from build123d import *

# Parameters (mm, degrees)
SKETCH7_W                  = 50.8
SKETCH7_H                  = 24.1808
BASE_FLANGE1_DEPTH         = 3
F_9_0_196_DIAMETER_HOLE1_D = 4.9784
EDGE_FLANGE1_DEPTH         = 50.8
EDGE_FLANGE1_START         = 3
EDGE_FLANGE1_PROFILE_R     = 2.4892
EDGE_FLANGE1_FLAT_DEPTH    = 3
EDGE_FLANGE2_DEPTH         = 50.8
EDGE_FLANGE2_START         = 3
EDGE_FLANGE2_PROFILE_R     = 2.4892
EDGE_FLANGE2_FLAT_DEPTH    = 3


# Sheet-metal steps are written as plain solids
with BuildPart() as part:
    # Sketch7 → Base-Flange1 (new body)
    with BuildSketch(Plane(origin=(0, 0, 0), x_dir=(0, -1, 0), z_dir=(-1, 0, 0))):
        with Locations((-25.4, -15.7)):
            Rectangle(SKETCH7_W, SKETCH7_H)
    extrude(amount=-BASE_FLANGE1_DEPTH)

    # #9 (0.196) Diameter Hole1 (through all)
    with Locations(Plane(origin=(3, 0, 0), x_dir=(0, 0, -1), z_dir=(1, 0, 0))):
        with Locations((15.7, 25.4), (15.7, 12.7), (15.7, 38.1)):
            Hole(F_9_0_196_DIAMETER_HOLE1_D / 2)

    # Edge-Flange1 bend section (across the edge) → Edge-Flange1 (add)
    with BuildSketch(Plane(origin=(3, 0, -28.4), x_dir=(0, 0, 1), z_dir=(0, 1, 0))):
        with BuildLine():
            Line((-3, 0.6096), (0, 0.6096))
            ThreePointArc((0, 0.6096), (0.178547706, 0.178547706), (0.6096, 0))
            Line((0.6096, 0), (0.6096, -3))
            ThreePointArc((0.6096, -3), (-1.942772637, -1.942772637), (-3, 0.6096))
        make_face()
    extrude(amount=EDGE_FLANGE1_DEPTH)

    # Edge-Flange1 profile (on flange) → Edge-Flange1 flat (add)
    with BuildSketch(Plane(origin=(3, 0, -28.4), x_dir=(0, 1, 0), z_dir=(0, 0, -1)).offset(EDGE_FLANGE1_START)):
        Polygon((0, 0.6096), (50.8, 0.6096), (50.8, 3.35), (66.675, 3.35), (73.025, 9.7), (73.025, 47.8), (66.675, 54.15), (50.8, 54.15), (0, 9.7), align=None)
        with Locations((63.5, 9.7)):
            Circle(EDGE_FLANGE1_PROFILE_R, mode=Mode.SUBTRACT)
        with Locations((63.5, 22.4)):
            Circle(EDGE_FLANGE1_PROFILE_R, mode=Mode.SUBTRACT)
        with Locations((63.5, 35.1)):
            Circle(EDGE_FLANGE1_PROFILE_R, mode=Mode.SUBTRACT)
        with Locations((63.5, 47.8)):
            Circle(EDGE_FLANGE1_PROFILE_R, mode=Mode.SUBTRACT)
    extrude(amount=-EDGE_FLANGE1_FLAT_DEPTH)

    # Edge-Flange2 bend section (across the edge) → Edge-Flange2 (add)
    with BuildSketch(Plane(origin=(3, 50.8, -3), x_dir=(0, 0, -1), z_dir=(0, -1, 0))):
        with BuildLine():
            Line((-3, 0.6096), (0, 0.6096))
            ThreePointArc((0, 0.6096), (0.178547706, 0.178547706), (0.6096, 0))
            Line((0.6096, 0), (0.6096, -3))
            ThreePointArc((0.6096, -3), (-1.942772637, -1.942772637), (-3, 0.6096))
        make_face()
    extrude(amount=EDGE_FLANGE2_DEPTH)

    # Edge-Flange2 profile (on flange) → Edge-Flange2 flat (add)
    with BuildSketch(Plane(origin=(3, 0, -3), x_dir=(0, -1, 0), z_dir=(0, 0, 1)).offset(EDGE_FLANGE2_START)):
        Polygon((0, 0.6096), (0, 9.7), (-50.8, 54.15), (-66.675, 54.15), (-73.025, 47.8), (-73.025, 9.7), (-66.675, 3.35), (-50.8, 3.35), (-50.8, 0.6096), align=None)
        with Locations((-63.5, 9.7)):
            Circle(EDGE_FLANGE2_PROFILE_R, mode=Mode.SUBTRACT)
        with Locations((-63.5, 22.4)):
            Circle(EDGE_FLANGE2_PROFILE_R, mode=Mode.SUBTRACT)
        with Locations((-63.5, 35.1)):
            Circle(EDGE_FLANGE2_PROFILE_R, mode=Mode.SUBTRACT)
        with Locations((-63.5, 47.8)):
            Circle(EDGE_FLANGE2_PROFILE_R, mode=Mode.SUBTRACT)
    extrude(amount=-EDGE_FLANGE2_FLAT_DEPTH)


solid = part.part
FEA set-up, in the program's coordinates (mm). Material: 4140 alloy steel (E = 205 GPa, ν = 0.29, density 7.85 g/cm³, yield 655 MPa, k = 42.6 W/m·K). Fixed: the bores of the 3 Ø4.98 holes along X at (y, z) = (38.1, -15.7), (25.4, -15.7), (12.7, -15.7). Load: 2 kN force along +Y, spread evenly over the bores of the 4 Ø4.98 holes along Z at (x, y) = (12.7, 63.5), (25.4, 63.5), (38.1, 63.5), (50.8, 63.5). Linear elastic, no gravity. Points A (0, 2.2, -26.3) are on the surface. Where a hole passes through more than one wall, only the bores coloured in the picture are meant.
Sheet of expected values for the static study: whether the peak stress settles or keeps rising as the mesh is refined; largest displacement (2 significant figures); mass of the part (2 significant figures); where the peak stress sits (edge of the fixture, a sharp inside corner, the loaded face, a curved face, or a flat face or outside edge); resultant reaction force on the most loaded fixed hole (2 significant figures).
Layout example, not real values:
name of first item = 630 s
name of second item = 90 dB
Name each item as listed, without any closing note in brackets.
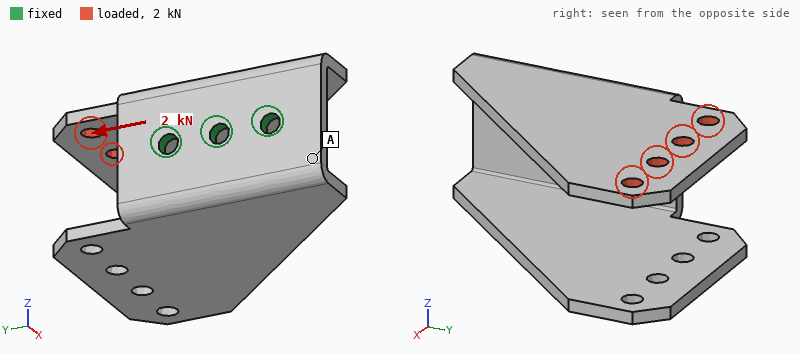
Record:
whether the peak stress settles or keeps rising as the mesh is refined = keeps rising
largest displacement = 0.52 mm
mass of the part = 160 g
where the peak stress sits = edge of the fixture
resultant reaction force on the most loaded fixed hole = 2.3 kN
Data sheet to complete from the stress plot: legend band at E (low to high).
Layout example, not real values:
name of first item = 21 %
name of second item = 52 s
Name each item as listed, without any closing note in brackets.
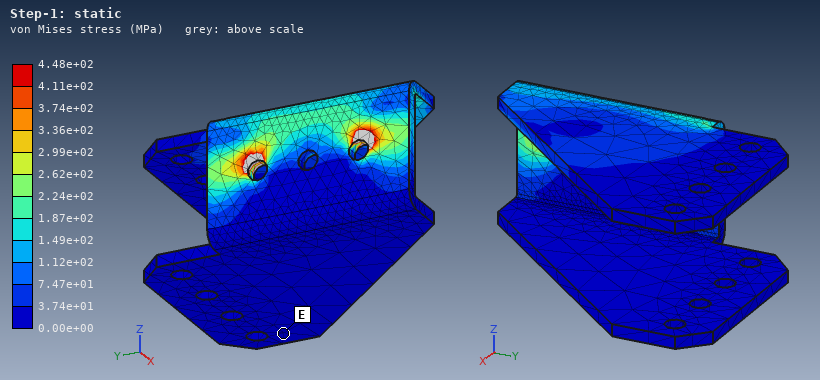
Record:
legend band at E = 0.00e+00 to 3.74e+01 MPa
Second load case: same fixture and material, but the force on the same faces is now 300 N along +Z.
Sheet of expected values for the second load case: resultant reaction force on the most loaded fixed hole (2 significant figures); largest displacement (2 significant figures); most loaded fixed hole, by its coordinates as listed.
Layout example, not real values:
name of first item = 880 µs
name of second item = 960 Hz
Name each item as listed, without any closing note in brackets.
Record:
resultant reaction force on the most loaded fixed hole = 570 N
largest displacement = 0.96 mm
most loaded fixed hole, by its coordinates as listed = (38.1, -15.7)
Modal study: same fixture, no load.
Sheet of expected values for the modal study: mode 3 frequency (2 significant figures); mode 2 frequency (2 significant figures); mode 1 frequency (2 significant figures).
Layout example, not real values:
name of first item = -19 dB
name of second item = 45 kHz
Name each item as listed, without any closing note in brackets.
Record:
mode 3 frequency = 1600 Hz
mode 2 frequency = 610 Hz
mode 1 frequency = 610 Hz
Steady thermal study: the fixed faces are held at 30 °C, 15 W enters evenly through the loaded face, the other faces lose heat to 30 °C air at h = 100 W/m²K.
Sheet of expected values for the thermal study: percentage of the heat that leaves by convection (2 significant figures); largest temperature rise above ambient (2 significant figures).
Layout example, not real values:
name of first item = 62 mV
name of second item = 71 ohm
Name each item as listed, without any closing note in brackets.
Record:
percentage of the heat that leaves by convection = 87 %
largest temperature rise above ambient = 47 K
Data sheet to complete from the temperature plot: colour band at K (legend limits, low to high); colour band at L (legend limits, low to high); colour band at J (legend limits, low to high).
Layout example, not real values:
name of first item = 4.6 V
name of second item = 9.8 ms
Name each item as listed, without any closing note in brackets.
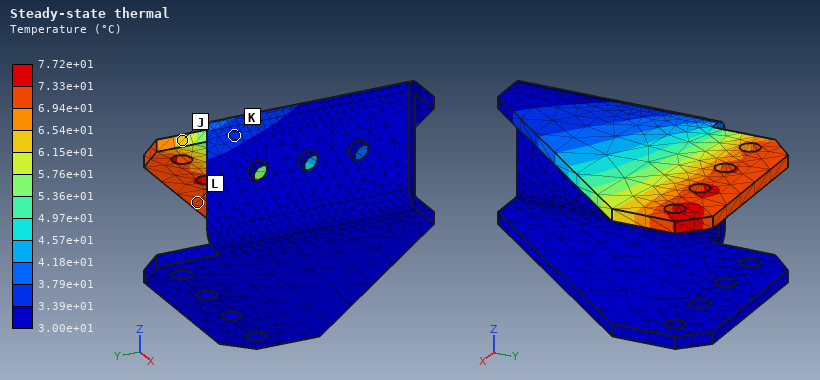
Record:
colour band at K = 3.39e+01 to 3.79e+01 °C
colour band at L = 6.94e+01 to 7.33e+01 °C
colour band at J = 6.15e+01 to 6.54e+01 °C
